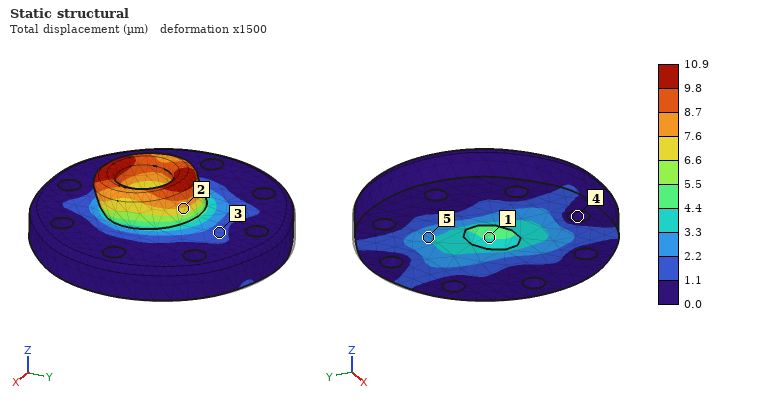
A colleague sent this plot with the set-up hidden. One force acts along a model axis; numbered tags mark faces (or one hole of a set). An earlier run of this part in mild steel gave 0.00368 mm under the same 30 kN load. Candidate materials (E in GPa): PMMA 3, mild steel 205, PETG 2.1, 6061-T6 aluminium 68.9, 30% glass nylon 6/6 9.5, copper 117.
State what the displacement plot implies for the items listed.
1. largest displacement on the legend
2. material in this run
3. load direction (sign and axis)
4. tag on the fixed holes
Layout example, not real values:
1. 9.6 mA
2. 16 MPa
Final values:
1. 10.9 µm
2. 6061-T6 aluminium
3. -Y
4. 4
